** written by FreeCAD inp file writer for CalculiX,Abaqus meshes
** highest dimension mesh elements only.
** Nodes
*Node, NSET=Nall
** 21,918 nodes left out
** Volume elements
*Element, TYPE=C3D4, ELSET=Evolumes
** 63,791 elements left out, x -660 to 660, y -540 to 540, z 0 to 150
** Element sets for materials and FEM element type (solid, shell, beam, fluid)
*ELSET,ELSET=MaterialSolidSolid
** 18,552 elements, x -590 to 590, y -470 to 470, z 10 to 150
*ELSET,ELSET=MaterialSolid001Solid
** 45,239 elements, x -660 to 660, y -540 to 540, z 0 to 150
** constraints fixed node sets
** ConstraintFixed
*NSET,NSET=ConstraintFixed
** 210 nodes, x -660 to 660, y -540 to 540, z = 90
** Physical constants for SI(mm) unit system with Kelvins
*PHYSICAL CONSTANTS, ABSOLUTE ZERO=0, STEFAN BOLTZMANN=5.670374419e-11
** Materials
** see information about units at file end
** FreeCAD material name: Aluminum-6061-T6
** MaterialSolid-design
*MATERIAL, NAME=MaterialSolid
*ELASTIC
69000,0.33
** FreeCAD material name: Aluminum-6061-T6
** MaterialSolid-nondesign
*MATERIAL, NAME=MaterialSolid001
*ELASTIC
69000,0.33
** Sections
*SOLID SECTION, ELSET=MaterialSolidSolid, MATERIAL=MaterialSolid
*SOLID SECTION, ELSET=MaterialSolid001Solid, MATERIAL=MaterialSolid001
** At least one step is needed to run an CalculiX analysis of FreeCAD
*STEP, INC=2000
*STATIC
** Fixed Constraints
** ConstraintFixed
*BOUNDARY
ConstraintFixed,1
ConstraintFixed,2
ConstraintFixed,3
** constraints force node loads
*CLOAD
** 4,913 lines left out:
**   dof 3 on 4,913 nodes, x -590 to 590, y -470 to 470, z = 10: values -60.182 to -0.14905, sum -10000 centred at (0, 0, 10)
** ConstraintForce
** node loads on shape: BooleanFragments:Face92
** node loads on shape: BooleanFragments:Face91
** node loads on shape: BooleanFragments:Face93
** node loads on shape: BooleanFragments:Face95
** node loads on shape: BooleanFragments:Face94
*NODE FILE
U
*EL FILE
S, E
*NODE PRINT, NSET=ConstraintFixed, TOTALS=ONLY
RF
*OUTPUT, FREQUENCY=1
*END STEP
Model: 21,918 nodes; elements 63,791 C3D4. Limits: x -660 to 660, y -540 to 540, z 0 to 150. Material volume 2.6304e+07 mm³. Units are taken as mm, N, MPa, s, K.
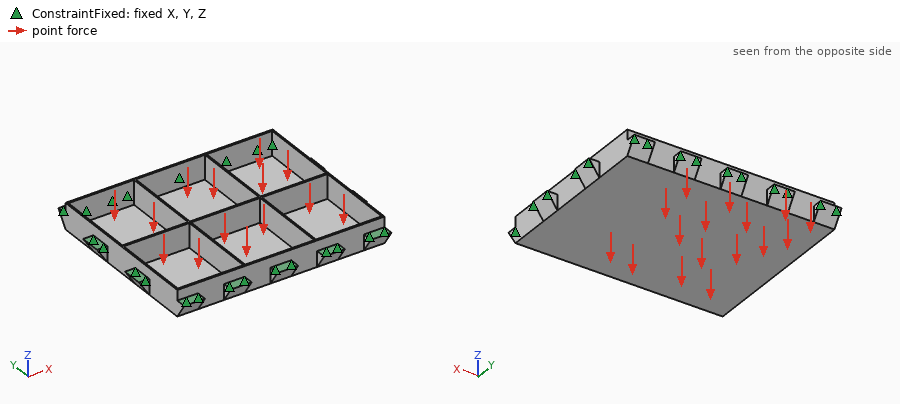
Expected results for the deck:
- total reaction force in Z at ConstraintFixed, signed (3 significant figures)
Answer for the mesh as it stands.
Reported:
10000 N
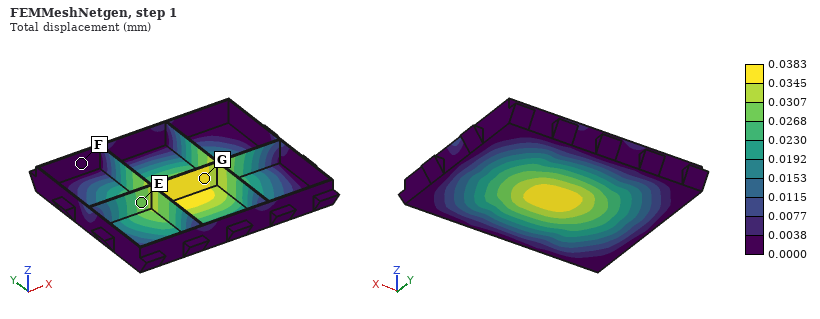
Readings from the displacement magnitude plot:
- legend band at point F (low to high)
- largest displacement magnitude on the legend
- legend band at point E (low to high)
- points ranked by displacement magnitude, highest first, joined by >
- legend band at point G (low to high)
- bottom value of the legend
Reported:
0.0000 to 0.0038 mm
0.0383 mm
0.0268 to 0.0307 mm
G > E > F
0.0345 to 0.0383 mm
0.0000 mm
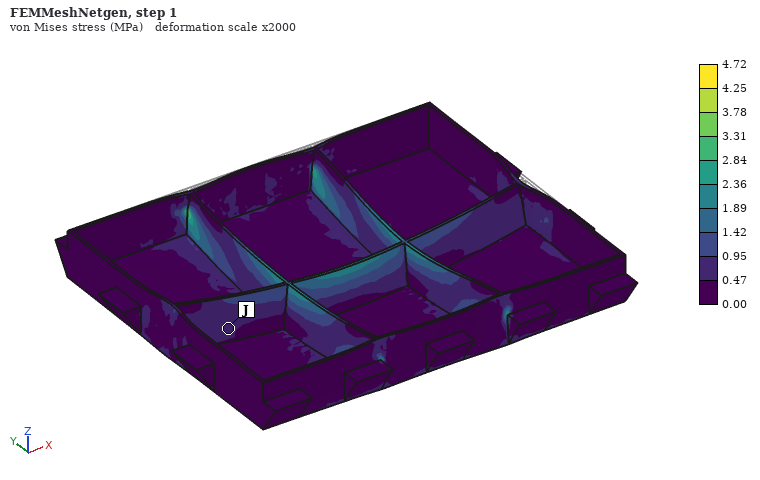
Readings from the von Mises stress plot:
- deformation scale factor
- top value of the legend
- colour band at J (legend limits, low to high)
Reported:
2000
4.72 MPa
0.47 to 0.95 MPa
